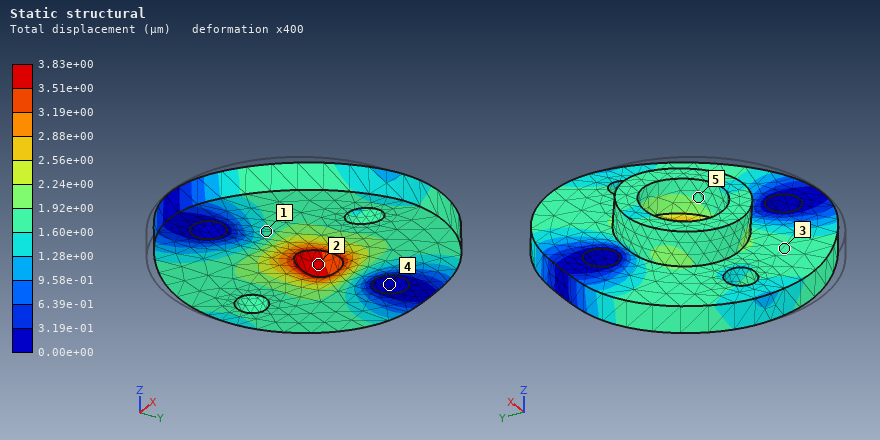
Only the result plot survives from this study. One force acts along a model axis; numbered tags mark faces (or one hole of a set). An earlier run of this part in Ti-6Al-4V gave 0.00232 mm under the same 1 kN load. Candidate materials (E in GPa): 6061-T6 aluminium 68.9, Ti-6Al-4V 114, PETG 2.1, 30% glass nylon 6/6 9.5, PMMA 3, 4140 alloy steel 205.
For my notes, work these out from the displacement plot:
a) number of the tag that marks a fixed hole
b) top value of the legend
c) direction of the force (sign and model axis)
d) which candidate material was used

4
3.83e+00 µm
+Y
6061-T6 aluminium
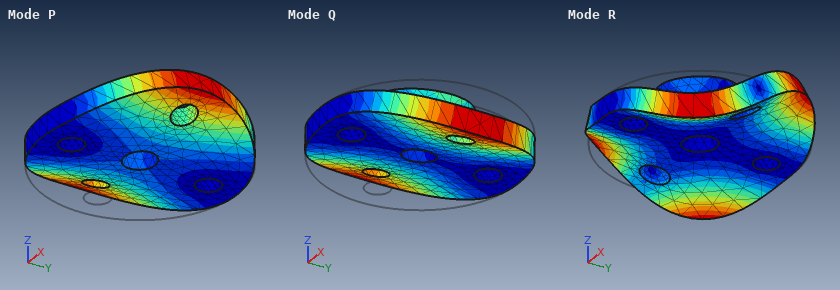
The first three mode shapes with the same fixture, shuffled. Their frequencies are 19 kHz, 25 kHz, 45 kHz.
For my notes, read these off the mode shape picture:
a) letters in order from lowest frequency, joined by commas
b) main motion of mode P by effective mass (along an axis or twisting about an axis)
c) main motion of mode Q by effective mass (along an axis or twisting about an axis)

Q, P, R
along Z
twisting about Y
